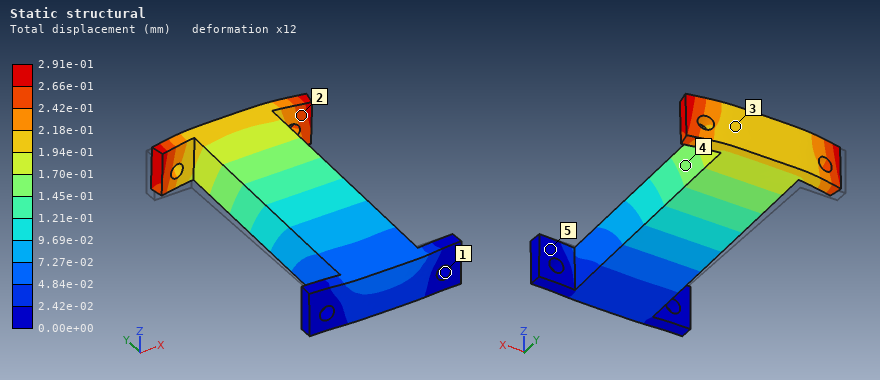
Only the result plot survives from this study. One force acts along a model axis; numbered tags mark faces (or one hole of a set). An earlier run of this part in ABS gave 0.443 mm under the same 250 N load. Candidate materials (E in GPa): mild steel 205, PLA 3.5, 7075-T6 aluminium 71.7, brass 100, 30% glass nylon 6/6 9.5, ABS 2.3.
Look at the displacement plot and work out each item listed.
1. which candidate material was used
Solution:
PLA
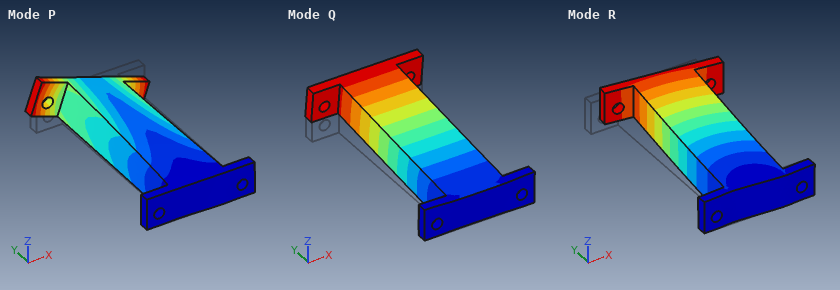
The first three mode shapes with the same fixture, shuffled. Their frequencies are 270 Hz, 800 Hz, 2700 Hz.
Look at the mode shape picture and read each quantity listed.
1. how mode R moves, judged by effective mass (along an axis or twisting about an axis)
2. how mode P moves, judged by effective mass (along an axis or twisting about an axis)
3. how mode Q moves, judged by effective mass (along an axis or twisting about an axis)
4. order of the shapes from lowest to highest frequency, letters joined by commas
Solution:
along X
twisting about Y
along Z
Q, R, P
